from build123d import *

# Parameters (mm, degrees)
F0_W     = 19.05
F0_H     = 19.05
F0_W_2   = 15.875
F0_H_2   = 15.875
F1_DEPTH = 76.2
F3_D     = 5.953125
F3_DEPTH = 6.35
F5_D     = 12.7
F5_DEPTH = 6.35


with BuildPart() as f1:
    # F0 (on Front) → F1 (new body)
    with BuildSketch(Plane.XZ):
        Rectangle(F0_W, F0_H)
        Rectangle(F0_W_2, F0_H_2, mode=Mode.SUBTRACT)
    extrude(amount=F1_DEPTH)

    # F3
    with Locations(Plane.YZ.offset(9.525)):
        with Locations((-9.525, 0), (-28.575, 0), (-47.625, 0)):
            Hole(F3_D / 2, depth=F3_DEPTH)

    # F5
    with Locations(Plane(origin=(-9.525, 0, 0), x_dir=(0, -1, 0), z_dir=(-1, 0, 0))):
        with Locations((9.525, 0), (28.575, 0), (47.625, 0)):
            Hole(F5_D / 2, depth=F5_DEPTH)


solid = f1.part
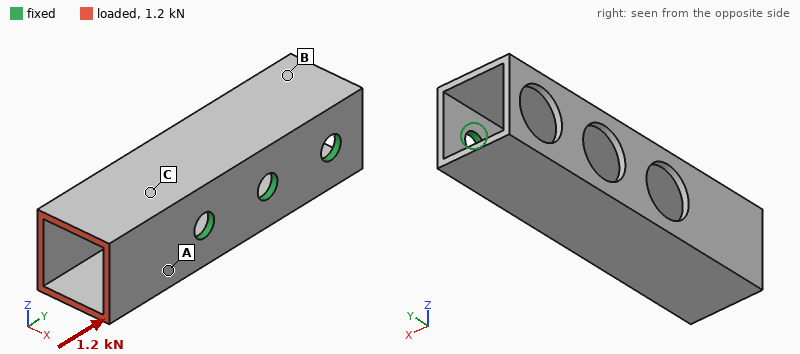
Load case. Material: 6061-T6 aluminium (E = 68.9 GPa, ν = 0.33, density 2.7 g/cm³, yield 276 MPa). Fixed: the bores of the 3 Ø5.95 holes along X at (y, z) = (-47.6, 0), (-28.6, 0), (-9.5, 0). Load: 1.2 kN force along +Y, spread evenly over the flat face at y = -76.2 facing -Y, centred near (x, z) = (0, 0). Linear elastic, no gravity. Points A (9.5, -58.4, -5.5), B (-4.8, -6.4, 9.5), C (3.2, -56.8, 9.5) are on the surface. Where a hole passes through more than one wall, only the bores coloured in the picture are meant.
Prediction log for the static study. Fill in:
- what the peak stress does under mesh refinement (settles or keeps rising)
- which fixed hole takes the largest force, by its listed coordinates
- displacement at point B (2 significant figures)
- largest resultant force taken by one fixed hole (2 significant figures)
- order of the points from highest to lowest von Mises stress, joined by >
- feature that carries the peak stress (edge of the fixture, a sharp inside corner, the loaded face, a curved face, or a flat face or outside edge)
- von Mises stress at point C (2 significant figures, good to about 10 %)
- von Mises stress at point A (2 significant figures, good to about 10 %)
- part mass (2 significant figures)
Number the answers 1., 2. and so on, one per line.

1. keeps rising
2. (-47.6, 0)
3. 24 µm
4. 650 N
5. A > C > B
6. edge of the fixture
7. 13 MPa
8. 25 MPa
9. 21 g
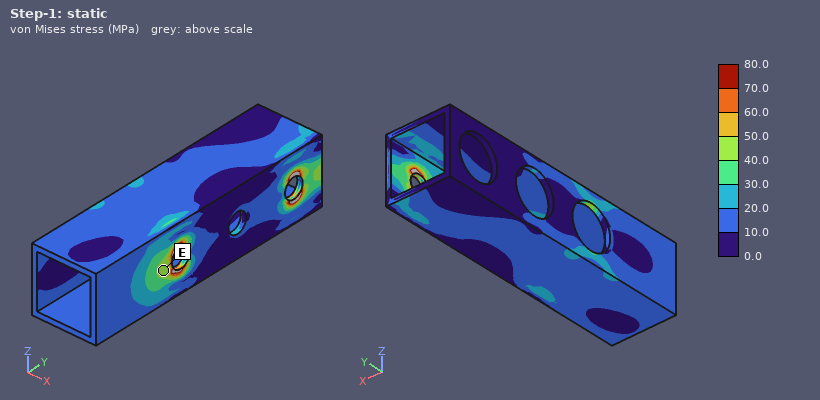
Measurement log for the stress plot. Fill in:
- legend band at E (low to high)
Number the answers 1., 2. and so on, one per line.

1. 40.0 to 50.0 MPa
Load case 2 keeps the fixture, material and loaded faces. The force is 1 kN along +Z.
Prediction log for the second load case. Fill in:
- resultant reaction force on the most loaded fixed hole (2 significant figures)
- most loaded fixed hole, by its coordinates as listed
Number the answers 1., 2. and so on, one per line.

1. 1.6 kN
2. (-47.6, 0)
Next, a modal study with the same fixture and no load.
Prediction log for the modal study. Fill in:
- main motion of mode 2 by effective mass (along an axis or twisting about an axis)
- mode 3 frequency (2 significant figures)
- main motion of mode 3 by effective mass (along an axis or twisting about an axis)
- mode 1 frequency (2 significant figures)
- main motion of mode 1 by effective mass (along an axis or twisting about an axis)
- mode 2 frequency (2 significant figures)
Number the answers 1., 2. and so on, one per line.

1. along X
2. 5800 Hz
3. twisting about X
4. 2300 Hz
5. along Z
6. 4100 Hz
